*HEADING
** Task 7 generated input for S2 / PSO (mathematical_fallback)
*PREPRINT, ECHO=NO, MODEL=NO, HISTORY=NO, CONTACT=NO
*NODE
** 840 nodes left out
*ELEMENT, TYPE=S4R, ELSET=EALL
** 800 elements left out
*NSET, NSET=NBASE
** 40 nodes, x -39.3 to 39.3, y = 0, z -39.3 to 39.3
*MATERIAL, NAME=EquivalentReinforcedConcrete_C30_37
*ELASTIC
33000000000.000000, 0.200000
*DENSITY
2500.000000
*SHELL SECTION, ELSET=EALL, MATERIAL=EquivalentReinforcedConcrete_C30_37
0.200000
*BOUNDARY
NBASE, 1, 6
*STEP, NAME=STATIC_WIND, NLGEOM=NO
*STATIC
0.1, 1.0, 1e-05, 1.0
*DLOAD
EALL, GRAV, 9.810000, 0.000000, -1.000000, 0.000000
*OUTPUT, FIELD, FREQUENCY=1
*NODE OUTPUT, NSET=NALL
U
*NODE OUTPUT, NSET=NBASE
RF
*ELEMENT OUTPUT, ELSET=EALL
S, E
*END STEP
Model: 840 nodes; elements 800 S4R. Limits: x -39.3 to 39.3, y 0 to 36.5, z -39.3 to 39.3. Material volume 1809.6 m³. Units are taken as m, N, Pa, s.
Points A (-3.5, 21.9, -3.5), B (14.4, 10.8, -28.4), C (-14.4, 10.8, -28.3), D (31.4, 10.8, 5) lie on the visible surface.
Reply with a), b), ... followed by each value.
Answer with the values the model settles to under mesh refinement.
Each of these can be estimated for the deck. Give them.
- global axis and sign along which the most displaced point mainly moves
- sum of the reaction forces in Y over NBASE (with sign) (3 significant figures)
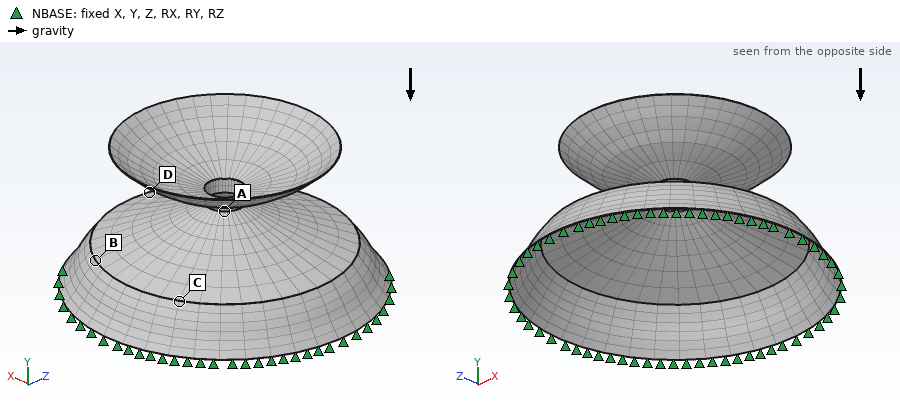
a) -Y
b) 4.44e+07 N
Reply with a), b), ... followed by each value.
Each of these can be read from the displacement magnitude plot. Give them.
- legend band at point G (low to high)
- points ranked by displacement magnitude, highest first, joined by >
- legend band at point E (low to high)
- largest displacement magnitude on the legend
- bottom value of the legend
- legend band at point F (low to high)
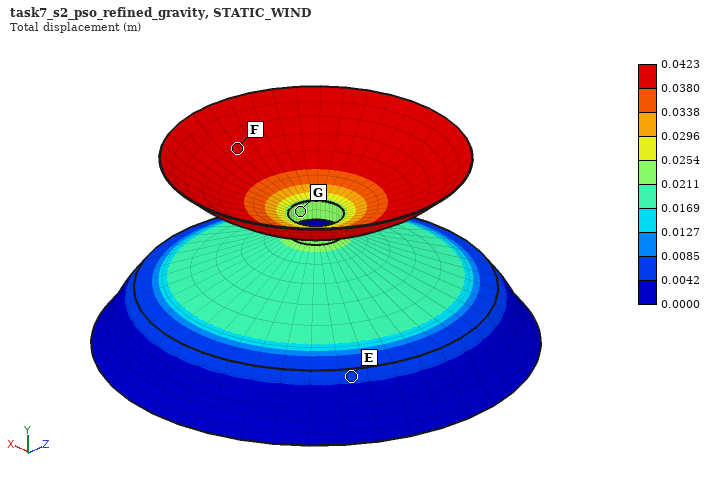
a) 0.0211 to 0.0254 m
b) F > G > E
c) 0.0042 to 0.0085 m
d) 0.0423 m
e) 0.0000 m
f) 0.0380 to 0.0423 m
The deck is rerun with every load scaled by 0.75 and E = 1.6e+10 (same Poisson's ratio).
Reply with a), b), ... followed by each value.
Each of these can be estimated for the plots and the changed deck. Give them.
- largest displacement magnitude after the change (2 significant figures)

a) 0.065 m
